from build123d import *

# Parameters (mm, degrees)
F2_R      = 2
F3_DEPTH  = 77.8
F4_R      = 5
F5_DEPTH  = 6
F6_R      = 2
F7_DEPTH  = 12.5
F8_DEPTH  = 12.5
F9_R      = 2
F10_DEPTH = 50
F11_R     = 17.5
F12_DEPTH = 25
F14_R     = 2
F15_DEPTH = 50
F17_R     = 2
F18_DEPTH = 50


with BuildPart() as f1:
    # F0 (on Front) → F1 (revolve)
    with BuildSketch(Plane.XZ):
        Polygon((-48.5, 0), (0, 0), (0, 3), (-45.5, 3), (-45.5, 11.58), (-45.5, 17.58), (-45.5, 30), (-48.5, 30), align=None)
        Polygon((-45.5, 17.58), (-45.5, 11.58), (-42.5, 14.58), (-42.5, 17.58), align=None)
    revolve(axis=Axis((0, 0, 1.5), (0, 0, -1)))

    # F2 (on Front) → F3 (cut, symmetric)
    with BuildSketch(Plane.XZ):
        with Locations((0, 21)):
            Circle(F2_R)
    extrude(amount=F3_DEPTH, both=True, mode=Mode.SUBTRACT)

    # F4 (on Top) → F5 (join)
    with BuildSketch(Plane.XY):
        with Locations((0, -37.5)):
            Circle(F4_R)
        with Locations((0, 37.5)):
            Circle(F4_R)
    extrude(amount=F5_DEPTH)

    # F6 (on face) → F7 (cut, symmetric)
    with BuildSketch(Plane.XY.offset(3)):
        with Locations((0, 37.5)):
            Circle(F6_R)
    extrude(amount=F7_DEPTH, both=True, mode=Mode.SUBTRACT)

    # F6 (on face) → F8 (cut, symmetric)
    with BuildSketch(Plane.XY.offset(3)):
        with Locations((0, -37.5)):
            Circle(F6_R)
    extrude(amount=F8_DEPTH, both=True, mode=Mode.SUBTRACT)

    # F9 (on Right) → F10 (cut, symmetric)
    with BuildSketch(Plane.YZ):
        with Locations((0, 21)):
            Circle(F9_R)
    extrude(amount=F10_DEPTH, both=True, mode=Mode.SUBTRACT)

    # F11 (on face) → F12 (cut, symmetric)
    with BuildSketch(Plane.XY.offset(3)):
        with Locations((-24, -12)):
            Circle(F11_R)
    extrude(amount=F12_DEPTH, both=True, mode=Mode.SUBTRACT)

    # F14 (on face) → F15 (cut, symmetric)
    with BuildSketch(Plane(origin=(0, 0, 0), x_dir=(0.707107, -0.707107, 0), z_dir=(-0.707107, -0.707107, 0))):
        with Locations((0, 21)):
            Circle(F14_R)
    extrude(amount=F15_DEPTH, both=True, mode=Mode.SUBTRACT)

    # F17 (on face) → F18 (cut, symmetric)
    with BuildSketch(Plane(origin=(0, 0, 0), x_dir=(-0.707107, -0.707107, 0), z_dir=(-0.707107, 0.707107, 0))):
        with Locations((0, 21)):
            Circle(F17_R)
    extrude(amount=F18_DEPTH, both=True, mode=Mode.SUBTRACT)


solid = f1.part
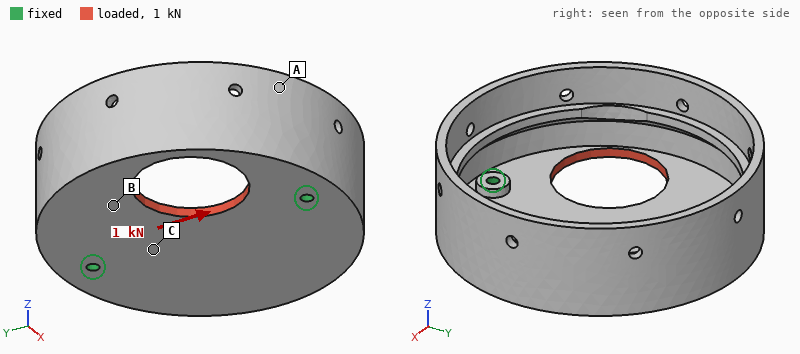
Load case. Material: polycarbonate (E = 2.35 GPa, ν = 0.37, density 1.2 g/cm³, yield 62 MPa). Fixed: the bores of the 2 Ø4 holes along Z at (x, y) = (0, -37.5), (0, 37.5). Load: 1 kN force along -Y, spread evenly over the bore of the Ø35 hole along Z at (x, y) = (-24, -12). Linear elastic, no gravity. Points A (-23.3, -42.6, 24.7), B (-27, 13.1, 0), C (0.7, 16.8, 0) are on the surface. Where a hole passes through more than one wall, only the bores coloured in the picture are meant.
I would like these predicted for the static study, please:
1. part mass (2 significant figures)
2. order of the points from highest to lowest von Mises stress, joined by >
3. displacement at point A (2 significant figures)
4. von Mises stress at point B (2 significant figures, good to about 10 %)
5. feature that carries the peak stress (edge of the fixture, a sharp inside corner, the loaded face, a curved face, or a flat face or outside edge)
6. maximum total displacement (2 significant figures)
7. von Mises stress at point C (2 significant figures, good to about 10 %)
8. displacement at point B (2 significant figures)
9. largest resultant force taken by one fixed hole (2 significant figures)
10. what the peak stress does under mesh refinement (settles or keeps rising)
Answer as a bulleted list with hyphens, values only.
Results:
- 56 g
- B > C > A
- 0.28 mm
- 7.7 MPa
- edge of the fixture
- 0.51 mm
- 4.2 MPa
- 0.24 mm
- 590 N
- keeps rising
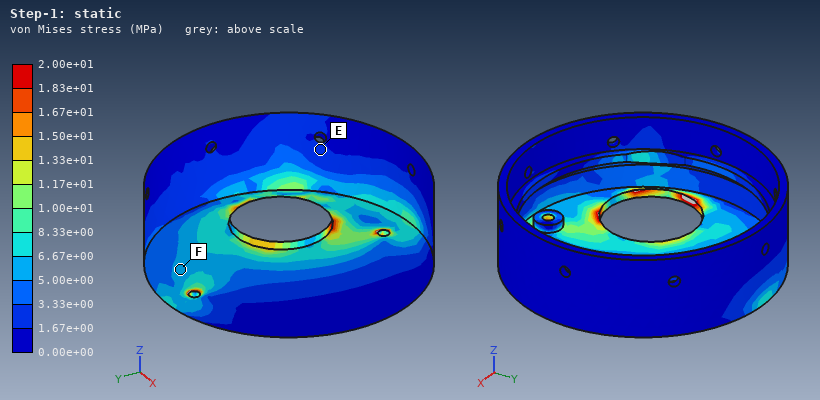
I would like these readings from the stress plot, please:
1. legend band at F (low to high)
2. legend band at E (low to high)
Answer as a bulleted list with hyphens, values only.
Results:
- 5.00e+00 to 6.67e+00 MPa
- 1.67e+00 to 3.33e+00 MPa
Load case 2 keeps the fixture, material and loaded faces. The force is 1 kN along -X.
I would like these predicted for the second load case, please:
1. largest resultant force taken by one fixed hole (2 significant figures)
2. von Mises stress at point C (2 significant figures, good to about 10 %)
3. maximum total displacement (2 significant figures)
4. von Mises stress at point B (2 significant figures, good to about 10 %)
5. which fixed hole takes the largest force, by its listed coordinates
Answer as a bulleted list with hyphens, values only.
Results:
- 660 N
- 2.7 MPa
- 0.37 mm
- 4.9 MPa
- (0, -37.5)
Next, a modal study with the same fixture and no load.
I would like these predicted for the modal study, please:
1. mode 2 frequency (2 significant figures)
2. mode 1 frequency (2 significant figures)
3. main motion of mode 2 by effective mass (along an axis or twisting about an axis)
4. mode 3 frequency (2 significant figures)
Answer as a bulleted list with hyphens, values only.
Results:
- 490 Hz
- 260 Hz
- along Z
- 590 Hz
